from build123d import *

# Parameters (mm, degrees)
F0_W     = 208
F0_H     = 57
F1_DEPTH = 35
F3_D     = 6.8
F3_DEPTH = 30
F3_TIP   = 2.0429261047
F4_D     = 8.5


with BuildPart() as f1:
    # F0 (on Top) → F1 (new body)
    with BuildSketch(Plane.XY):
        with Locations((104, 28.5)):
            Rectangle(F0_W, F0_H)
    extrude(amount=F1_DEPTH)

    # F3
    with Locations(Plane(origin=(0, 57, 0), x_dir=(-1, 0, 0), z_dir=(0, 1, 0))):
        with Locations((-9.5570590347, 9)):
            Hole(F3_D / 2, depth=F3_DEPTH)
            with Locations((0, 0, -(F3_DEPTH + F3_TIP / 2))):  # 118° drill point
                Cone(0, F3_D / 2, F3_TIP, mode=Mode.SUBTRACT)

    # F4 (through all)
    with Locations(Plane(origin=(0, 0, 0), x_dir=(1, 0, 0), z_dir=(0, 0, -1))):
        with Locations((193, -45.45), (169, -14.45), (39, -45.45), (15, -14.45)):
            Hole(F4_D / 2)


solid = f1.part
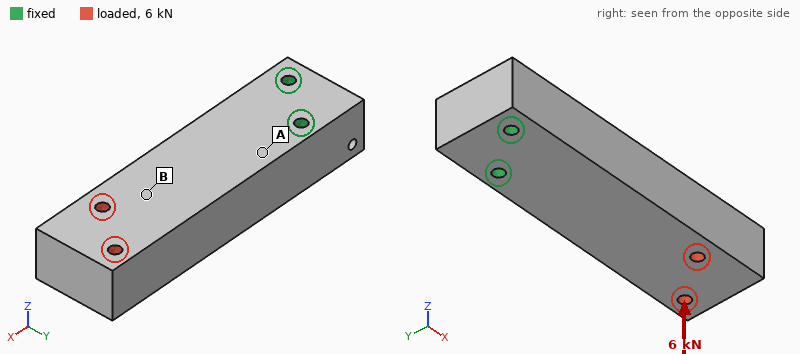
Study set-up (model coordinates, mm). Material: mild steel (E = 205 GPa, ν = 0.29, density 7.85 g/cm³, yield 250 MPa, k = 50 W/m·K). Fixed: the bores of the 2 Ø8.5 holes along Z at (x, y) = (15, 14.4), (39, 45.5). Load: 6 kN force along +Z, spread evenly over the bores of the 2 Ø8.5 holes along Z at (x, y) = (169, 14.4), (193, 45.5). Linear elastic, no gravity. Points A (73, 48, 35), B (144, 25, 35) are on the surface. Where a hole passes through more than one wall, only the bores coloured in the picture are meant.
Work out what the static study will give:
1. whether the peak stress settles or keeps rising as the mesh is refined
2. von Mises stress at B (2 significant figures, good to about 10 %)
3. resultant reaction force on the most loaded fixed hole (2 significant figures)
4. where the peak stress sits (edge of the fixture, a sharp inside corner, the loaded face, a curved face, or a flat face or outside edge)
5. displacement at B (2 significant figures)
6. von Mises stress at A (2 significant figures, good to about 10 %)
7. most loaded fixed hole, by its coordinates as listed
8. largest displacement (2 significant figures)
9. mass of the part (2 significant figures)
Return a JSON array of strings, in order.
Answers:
["keeps rising", "19 MPa", "9.7 kN", "edge of the fixture", "0.11 mm", "59 MPa", "(39, 45.5)", "0.21 mm", "3.2 kg"]
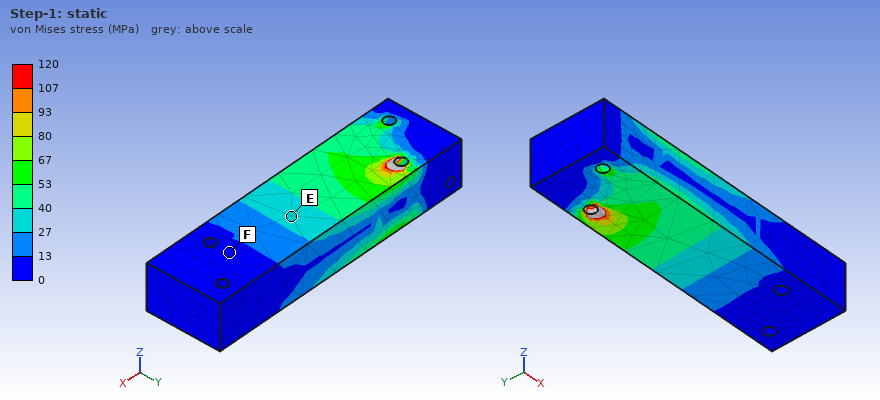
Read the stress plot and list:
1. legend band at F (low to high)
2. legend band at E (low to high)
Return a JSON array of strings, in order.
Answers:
["0 to 13 MPa", "27 to 40 MPa"]
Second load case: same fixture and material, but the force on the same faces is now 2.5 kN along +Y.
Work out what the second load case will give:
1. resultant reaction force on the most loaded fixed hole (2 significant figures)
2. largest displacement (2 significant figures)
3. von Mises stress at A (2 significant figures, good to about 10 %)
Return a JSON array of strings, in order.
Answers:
["9.6 kN", "38 µm", "9.6 MPa"]
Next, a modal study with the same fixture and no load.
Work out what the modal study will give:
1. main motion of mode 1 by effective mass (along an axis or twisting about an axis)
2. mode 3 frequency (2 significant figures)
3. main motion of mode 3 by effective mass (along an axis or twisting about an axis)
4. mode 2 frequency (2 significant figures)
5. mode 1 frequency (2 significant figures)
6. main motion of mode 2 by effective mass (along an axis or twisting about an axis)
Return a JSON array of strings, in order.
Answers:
["along Z", "3800 Hz", "twisting about X", "1400 Hz", "920 Hz", "along Y"]
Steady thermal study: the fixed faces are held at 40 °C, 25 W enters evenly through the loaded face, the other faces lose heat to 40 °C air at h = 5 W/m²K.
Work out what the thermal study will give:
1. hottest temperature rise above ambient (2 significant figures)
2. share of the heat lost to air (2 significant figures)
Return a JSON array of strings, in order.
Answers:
["36 K", "14 %"]
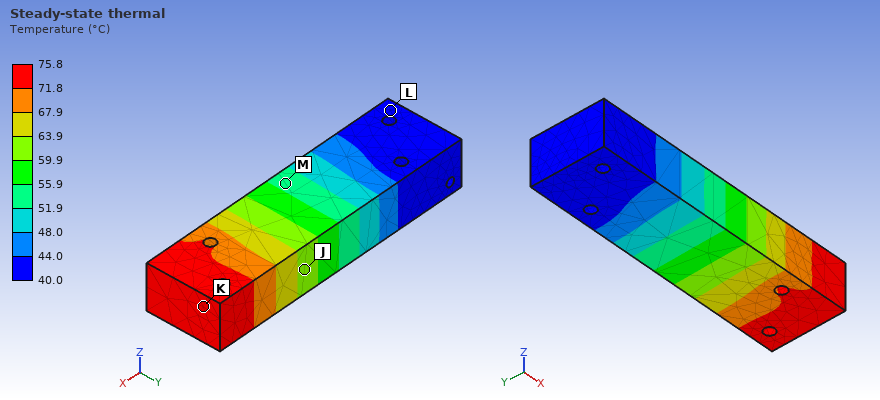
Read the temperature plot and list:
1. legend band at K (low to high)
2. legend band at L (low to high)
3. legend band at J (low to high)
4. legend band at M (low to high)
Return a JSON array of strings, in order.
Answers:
["71.8 to 75.8 °C", "40.0 to 44.0 °C", "59.9 to 63.9 °C", "51.9 to 55.9 °C"]
